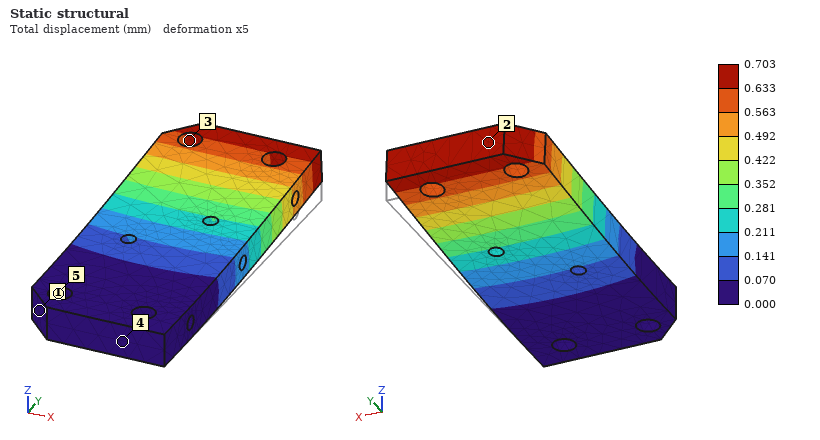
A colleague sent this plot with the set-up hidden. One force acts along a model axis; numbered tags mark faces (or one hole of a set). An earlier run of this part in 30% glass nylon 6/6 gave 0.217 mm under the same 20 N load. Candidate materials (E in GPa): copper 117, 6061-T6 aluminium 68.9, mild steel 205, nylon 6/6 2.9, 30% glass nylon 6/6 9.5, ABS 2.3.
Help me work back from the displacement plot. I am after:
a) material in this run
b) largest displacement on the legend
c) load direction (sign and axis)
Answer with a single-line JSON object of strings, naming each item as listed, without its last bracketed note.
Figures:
{"material in this run": "nylon 6/6", "largest displacement on the legend": "0.703 mm", "load direction": "+Z"}
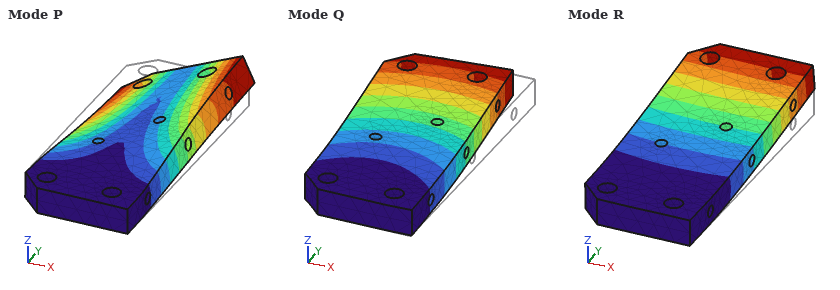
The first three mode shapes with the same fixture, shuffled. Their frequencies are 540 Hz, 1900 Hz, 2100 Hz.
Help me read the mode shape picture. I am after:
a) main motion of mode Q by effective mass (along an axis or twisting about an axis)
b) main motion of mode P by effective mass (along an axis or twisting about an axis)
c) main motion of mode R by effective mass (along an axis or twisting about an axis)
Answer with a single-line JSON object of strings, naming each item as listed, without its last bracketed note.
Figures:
{"main motion of mode Q by effective mass": "along X", "main motion of mode P by effective mass": "twisting about Y", "main motion of mode R by effective mass": "along Z"}
